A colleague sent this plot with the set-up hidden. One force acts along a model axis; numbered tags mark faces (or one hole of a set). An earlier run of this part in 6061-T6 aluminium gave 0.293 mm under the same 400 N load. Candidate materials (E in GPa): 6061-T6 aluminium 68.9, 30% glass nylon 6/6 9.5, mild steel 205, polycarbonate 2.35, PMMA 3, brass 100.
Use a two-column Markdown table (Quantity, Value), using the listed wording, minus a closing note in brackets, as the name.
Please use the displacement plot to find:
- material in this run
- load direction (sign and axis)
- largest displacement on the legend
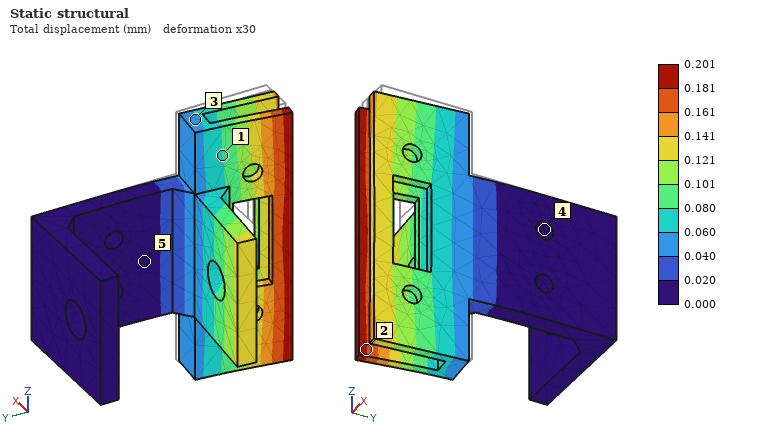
| Quantity | Value |
|---|---|
| material in this run | brass |
| load direction | -X |
| largest displacement on the legend | 0.201 mm |
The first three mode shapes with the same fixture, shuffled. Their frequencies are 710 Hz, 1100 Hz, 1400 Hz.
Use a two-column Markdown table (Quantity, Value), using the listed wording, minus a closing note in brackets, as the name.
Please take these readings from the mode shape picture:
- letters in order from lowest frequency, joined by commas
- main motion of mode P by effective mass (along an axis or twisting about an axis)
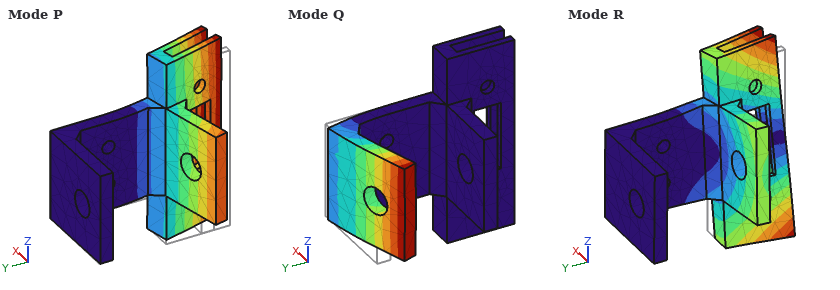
| Quantity | Value |
|---|---|
| letters in order from lowest frequency, joined by commas | P, R, Q |
| main motion of mode P by effective mass | along X |
